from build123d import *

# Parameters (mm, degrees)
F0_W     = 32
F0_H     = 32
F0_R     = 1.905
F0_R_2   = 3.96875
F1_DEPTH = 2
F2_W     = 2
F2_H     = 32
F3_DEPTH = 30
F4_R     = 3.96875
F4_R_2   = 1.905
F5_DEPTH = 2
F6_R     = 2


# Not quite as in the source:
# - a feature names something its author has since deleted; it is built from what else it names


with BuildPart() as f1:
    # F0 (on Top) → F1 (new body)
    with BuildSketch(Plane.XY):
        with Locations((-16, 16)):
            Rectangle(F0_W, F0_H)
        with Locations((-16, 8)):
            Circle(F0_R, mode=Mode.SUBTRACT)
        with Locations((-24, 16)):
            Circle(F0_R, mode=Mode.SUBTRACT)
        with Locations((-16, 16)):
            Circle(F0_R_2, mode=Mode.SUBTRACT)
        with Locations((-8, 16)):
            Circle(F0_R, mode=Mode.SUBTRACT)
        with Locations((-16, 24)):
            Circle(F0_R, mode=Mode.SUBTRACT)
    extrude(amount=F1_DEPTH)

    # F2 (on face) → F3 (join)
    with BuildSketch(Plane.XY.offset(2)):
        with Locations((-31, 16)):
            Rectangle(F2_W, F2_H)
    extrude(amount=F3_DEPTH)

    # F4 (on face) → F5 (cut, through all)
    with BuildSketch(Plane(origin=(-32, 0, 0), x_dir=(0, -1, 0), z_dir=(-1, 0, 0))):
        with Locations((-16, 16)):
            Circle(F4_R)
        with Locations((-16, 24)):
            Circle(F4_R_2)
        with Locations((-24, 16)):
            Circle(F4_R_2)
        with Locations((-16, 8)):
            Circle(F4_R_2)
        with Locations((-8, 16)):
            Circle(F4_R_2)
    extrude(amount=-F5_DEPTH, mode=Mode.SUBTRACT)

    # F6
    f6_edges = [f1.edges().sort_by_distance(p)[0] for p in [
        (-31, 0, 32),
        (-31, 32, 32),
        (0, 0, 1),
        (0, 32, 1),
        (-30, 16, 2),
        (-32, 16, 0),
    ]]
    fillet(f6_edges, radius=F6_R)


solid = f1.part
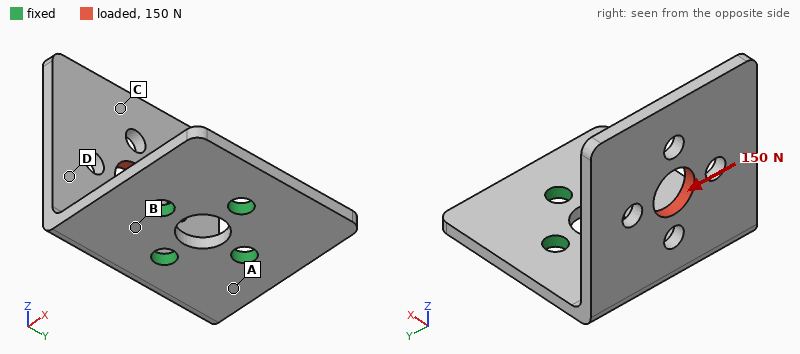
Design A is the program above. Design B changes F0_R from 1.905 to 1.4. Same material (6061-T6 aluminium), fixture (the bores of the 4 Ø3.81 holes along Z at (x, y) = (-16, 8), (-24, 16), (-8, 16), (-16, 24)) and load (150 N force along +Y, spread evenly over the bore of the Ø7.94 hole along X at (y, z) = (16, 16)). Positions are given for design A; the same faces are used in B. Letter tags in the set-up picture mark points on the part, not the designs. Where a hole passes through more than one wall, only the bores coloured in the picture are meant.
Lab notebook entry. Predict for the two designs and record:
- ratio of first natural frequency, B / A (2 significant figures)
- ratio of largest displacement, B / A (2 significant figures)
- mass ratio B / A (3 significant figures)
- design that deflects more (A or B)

0.98
1.1
1.01
B
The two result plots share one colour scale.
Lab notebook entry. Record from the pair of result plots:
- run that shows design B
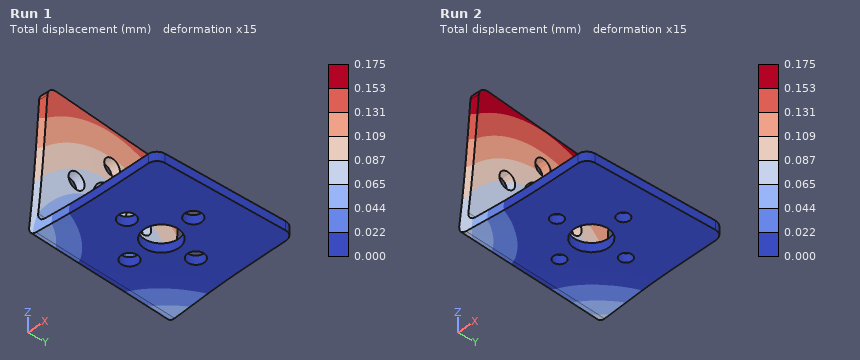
Run 2
